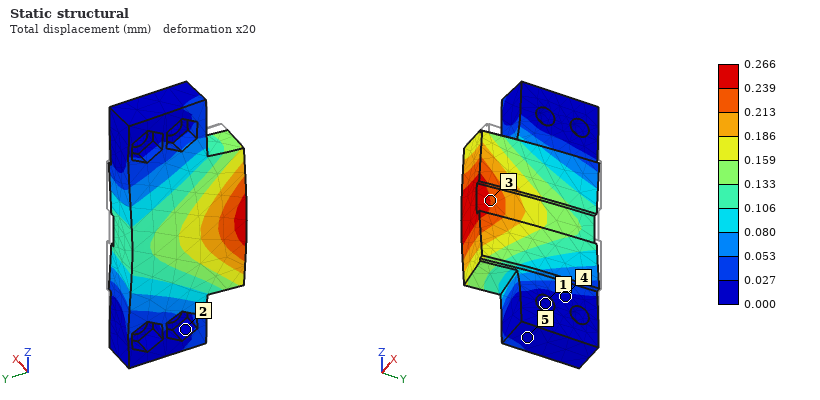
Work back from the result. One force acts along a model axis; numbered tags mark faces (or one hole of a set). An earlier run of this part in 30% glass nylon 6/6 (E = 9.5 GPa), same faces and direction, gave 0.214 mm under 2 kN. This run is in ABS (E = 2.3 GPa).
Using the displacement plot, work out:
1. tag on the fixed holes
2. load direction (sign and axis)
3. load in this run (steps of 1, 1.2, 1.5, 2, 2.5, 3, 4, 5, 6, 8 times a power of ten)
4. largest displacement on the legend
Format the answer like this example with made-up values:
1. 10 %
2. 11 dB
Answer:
1. 1
2. -X
3. 600 N
4. 0.266 mm
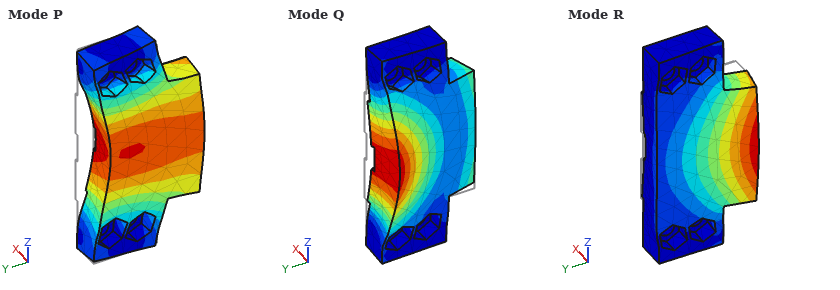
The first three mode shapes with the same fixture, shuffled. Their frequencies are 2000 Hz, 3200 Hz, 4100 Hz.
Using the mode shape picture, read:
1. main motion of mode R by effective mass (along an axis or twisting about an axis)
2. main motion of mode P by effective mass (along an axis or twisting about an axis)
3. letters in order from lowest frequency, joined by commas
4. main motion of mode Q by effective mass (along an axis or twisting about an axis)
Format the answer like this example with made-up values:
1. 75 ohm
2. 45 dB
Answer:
1. along X
2. along Y
3. R, Q, P
4. along X
